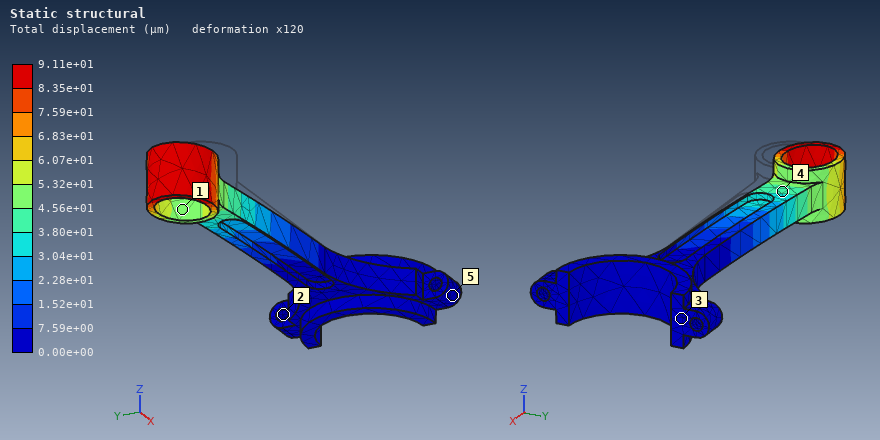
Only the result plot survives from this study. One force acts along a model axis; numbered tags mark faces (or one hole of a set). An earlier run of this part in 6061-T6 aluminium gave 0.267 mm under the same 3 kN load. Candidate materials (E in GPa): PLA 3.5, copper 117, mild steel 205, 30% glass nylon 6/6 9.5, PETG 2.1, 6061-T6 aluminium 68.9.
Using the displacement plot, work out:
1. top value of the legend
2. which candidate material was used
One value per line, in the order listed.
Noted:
9.11e+01 µm
mild steel
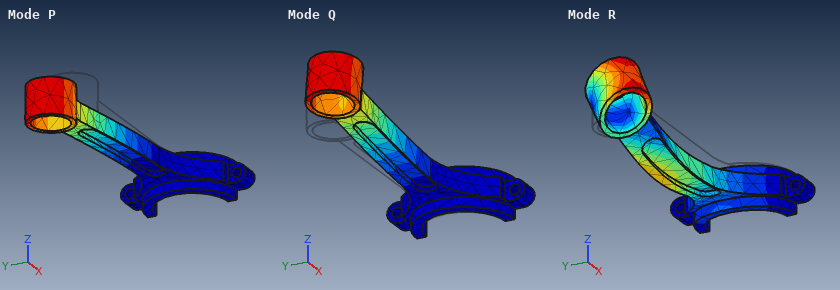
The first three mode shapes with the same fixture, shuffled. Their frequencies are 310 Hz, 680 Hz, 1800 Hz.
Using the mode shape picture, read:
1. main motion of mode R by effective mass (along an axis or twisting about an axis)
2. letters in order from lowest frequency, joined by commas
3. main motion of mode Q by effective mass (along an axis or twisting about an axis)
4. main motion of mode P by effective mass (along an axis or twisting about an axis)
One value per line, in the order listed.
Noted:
along Z
Q, P, R
along Z
along Y
